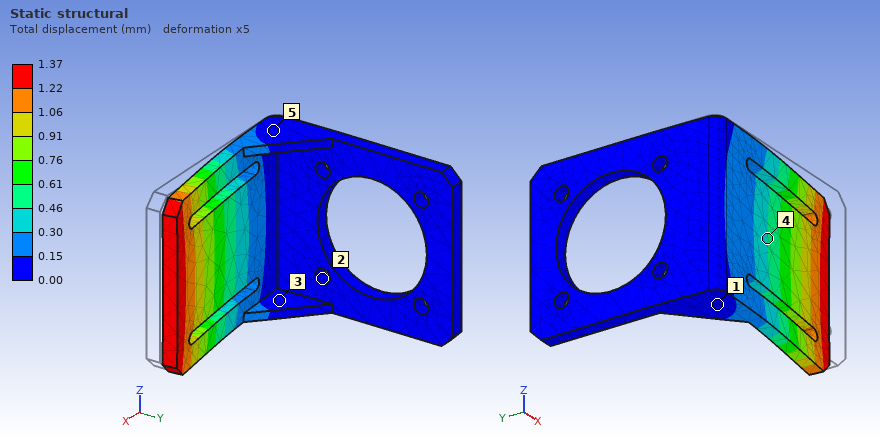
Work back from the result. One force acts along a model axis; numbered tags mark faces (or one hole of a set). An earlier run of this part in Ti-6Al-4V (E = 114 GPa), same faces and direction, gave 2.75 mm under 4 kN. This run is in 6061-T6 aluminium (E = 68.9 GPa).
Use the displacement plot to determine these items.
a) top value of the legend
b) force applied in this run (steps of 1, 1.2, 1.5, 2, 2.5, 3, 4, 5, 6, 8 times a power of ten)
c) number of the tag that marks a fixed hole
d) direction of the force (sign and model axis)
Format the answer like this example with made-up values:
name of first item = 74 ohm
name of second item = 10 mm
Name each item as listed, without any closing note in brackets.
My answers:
top value of the legend = 1.37 mm
force applied in this run = 1.2 kN
number of the tag that marks a fixed hole = 2
direction of the force = +Y
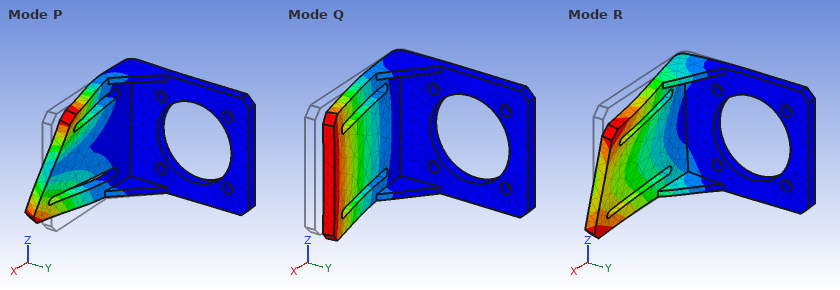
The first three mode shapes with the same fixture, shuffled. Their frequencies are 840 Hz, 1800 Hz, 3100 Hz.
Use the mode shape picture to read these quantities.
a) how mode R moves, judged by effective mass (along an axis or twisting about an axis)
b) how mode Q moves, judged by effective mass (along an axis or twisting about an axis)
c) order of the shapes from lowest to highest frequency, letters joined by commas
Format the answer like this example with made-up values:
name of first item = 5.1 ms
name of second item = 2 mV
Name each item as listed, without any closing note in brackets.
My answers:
how mode R moves, judged by effective mass = along Z
how mode Q moves, judged by effective mass = along Y
order of the shapes from lowest to highest frequency, letters joined by commas = Q, R, P
